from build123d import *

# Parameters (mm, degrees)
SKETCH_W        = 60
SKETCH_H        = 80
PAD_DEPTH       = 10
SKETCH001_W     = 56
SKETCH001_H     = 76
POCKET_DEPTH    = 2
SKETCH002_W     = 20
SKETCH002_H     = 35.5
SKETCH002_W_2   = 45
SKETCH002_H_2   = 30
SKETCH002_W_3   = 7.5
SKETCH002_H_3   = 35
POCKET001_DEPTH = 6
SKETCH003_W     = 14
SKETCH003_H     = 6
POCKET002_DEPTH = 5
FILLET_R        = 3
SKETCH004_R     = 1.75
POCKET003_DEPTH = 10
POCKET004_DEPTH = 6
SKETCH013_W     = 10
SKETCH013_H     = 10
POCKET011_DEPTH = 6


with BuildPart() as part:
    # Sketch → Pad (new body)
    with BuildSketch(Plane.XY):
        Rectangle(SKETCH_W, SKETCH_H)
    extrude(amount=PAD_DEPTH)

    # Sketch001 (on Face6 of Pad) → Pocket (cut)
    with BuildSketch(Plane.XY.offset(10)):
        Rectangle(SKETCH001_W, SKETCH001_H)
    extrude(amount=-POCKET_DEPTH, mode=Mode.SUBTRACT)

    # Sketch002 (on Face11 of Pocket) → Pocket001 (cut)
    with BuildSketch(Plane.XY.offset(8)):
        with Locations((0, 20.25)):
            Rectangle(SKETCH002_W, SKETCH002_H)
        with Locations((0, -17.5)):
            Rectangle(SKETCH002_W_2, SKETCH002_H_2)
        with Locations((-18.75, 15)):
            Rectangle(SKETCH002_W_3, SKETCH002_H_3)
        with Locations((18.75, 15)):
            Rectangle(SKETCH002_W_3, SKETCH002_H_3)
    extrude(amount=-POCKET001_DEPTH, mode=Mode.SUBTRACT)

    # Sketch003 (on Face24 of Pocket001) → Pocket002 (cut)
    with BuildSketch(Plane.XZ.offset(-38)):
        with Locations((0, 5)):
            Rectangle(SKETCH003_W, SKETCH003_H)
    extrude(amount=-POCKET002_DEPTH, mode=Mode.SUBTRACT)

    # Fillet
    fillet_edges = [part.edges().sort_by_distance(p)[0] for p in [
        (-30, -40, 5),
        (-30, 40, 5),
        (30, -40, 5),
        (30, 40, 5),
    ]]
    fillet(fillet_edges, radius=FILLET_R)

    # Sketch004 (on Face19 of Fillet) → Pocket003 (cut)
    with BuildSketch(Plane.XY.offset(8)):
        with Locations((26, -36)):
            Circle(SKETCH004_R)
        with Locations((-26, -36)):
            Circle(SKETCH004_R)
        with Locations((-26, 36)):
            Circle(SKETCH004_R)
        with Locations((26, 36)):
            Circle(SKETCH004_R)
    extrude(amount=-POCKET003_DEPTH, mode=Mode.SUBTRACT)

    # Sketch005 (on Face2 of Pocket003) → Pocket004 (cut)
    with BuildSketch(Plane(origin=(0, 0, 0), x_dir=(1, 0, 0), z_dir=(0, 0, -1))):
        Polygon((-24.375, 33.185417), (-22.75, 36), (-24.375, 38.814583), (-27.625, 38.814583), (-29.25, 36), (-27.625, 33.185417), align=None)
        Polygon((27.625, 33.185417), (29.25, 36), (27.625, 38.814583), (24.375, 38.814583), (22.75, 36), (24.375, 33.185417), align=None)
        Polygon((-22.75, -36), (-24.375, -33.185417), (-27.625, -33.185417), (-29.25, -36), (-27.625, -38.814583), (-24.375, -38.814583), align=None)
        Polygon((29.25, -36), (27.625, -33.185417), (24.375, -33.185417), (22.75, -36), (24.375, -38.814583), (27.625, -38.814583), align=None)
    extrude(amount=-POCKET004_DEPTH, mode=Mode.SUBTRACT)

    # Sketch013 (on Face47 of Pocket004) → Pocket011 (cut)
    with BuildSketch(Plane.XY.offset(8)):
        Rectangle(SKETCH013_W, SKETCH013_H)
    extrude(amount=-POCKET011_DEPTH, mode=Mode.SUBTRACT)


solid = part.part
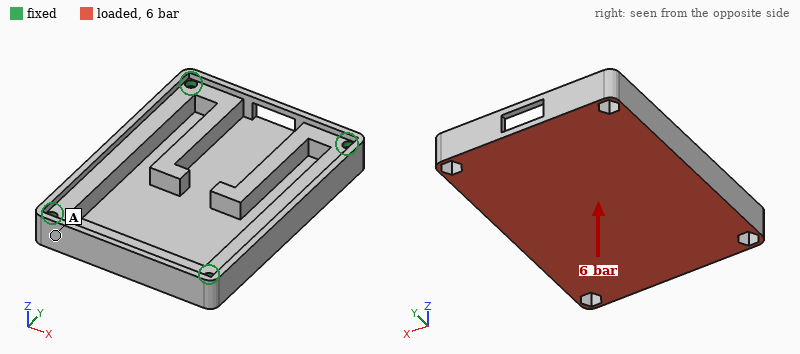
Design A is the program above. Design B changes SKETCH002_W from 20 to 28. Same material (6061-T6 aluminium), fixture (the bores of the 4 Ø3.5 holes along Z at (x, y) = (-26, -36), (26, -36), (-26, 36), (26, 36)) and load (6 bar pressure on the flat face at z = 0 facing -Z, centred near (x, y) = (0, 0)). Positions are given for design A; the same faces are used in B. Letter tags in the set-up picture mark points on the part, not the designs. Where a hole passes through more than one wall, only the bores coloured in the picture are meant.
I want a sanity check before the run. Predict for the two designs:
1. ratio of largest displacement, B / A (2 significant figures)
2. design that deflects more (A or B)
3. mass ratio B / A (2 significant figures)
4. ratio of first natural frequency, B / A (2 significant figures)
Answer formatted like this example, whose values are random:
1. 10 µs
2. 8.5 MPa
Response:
1. 1.2
2. B
3. 0.92
4. 0.97
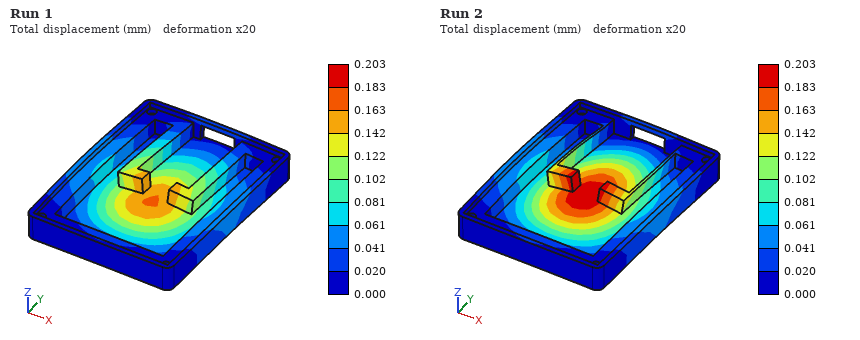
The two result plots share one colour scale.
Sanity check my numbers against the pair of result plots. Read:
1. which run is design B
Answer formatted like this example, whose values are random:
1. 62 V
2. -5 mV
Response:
1. Run 2
